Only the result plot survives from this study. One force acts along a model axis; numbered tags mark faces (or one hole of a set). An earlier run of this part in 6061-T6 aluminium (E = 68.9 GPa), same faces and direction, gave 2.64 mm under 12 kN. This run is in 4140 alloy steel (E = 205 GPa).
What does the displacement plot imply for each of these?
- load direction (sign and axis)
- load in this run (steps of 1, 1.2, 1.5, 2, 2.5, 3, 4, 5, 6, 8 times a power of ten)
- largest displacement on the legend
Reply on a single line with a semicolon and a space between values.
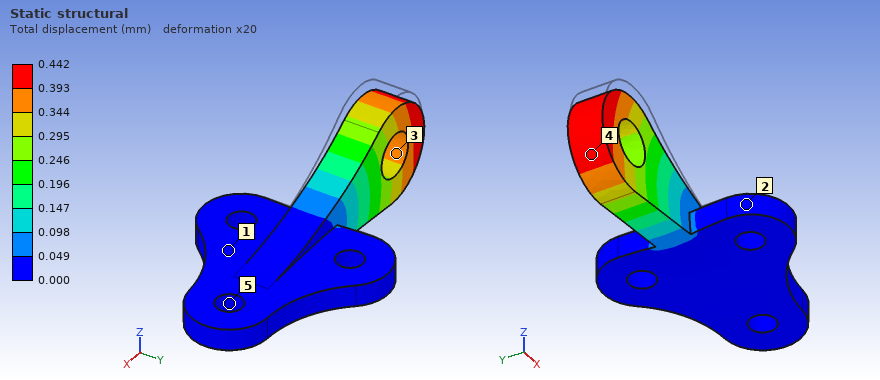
-Z; 6 kN; 0.442 mm
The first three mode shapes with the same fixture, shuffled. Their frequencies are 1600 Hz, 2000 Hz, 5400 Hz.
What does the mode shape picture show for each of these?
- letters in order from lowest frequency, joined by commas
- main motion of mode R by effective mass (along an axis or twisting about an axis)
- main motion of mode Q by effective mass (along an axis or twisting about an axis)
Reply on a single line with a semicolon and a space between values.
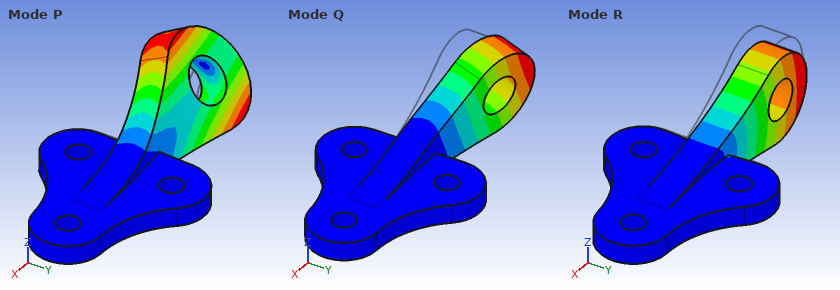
R, Q, P; along Z; along Y
